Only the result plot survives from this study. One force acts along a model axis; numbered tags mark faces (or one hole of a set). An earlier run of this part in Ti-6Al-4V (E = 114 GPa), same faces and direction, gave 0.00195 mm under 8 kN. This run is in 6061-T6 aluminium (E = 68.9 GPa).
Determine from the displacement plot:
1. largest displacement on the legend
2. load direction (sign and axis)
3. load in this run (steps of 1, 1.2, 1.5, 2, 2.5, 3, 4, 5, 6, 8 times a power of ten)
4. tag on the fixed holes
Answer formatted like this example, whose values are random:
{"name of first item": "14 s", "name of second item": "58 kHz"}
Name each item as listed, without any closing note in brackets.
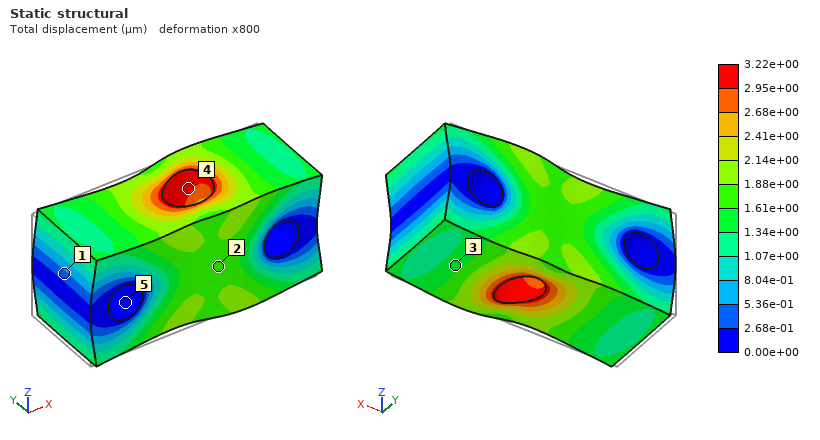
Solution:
{"largest displacement on the legend": "3.22e+00 µm", "load direction": "+X", "load in this run": "8 kN", "tag on the fixed holes": "5"}
